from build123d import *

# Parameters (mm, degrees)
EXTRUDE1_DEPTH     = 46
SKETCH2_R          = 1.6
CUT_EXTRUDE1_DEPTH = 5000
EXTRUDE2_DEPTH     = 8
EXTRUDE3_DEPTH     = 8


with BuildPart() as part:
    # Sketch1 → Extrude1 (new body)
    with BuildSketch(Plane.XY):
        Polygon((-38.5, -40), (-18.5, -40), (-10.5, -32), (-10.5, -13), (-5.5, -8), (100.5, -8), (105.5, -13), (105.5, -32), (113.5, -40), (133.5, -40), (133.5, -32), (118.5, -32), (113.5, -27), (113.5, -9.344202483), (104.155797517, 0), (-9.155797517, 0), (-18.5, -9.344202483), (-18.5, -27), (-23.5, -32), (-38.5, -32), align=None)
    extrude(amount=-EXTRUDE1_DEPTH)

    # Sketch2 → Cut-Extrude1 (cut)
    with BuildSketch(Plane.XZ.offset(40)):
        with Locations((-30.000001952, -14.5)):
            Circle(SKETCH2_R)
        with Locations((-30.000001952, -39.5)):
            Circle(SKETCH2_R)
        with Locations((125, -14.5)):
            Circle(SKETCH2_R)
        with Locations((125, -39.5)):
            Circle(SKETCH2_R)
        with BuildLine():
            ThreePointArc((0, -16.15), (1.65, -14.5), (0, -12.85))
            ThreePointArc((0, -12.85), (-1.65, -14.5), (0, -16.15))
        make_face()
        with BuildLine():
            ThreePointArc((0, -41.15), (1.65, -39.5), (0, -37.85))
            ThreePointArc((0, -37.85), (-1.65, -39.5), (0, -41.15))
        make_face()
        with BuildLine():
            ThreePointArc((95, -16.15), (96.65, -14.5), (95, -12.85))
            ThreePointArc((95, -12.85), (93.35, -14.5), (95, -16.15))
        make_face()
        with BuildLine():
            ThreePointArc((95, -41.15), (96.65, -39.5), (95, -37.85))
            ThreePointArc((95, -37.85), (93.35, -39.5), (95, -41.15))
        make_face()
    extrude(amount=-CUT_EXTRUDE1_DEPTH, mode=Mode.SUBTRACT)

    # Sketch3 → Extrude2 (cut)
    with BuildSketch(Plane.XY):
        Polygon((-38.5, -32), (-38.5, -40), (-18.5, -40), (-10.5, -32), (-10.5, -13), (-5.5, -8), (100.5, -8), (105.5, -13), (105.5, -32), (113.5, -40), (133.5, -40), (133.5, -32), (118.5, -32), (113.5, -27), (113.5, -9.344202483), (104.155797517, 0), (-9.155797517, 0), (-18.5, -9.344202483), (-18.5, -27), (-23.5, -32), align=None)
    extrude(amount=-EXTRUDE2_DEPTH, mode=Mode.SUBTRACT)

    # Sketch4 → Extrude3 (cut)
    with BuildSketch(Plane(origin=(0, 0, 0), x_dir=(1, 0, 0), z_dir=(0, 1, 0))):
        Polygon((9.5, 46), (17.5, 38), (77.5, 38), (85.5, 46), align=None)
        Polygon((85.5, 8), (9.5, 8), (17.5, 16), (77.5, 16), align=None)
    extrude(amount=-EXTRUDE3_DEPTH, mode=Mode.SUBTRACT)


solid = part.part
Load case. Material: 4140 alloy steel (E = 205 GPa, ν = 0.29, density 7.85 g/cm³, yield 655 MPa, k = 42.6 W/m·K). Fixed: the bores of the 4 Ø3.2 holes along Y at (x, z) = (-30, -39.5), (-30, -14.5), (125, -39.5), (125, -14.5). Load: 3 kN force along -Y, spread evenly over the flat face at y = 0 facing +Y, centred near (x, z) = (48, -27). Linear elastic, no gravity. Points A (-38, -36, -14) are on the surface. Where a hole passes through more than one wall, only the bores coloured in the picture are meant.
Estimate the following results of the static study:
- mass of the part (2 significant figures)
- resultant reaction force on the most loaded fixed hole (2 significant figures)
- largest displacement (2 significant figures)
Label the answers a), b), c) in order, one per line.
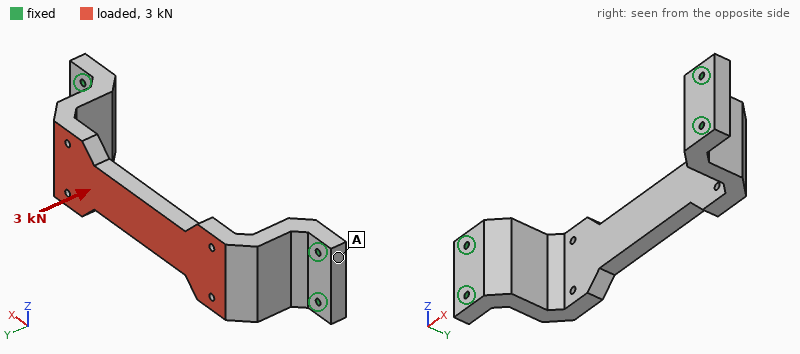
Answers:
a) 460 g
b) 1.1 kN
c) 63 µm
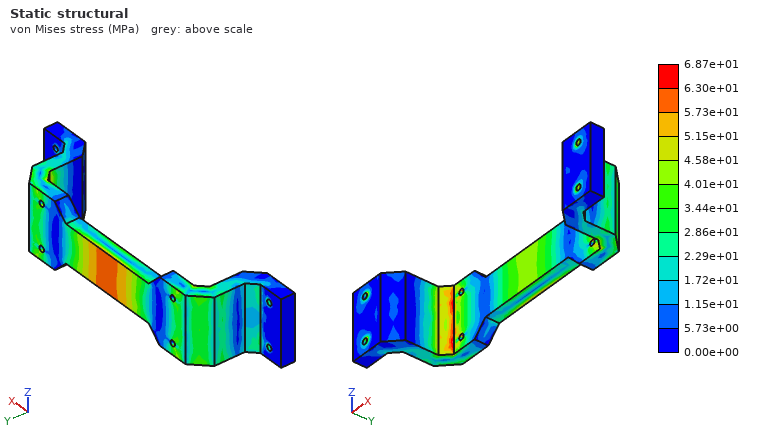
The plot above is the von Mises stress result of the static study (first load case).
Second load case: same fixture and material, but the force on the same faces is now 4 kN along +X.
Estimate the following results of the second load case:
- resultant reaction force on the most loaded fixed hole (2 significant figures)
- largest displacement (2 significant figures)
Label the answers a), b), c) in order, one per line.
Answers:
a) 1.1 kN
b) 65 µm
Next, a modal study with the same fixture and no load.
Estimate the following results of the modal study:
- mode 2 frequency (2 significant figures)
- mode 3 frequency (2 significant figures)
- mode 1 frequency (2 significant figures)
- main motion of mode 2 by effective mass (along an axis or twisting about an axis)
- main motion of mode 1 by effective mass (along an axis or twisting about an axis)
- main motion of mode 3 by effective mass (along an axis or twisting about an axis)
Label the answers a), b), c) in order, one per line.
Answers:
a) 2900 Hz
b) 3300 Hz
c) 2400 Hz
d) along Y
e) along X
f) along Z
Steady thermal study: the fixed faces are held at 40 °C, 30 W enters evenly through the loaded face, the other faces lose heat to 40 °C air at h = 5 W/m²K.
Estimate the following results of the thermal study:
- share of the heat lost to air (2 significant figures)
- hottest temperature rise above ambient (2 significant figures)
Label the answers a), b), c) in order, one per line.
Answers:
a) 9.2 %
b) 80 K
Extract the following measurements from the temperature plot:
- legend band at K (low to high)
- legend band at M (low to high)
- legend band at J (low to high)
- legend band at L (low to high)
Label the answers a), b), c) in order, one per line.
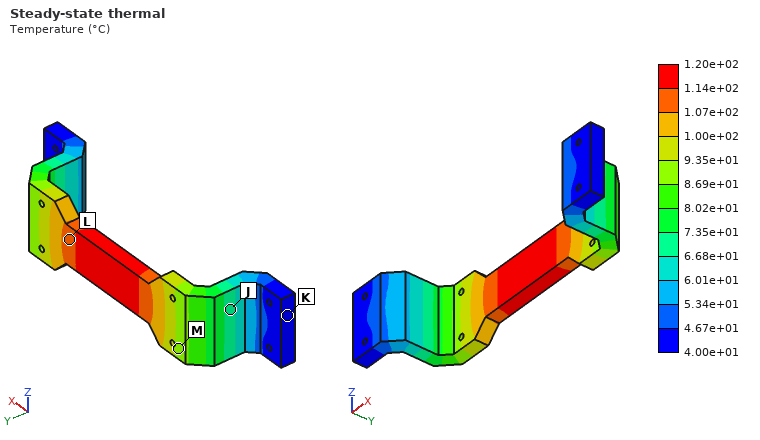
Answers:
a) 4.00e+01 to 4.67e+01 °C
b) 8.69e+01 to 9.35e+01 °C
c) 6.68e+01 to 7.35e+01 °C
d) 1.07e+02 to 1.14e+02 °C
